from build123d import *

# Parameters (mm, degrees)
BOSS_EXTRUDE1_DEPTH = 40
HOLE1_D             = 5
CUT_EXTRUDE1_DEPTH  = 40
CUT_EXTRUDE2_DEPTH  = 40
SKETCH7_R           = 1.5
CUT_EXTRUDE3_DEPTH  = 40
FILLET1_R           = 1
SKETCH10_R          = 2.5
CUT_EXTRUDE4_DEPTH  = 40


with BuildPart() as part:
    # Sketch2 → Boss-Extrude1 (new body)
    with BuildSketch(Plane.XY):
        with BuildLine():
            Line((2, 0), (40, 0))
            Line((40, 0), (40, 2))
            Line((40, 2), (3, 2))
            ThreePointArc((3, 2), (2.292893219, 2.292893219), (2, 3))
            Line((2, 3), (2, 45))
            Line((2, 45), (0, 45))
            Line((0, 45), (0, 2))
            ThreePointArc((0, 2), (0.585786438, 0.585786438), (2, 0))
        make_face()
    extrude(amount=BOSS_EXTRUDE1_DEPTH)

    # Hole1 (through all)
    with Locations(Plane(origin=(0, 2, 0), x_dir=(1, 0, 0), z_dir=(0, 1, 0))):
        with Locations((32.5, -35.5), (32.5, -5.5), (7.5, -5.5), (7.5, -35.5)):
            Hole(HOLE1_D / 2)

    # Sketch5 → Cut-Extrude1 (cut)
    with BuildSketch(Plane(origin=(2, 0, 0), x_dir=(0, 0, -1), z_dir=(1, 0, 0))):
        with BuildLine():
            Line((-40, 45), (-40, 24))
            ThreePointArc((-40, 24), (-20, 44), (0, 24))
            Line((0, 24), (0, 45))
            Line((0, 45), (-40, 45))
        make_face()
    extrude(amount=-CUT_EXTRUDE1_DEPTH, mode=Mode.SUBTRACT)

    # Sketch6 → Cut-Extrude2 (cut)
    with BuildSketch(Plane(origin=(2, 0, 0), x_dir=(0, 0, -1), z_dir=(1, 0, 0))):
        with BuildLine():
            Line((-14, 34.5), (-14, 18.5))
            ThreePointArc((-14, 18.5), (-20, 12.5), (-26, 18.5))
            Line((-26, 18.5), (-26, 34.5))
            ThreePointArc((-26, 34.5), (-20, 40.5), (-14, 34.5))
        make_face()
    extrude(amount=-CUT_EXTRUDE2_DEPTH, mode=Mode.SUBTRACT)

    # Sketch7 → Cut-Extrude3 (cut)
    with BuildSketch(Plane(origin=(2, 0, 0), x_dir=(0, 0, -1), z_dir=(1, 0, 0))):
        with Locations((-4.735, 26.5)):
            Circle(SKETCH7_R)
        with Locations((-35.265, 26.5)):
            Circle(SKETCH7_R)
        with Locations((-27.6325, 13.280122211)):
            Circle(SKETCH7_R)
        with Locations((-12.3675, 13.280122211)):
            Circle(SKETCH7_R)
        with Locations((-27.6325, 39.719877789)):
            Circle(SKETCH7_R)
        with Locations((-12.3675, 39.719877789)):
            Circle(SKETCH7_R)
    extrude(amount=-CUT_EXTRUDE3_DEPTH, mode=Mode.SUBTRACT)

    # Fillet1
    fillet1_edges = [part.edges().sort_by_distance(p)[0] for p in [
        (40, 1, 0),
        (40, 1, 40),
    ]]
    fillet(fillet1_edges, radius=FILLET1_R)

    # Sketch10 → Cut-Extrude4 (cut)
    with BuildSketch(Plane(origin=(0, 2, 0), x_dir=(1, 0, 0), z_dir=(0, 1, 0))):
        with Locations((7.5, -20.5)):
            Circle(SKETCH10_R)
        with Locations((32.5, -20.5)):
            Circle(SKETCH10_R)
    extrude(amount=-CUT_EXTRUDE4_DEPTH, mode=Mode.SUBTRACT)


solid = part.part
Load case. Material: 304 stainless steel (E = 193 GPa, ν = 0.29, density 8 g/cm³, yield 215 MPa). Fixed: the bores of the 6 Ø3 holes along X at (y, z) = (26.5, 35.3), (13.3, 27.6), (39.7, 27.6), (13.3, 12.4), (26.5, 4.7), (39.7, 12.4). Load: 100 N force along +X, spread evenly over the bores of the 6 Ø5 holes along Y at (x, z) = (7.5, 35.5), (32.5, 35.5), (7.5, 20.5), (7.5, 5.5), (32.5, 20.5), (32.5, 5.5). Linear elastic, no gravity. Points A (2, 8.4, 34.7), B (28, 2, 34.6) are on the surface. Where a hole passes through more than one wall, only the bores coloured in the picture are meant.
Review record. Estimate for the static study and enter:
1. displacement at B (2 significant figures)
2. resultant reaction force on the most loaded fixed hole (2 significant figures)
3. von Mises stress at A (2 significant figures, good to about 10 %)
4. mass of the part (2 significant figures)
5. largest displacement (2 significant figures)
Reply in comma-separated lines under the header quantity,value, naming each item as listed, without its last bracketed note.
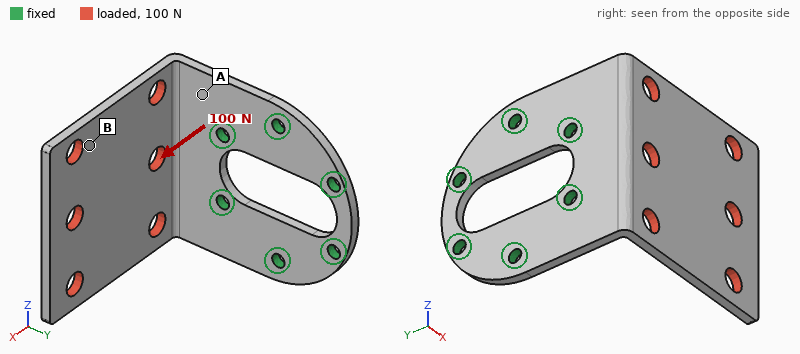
quantity,value
displacement at B,43 µm
resultant reaction force on the most loaded fixed hole,63 N
von Mises stress at A,24 MPa
mass of the part,42 g
largest displacement,62 µm
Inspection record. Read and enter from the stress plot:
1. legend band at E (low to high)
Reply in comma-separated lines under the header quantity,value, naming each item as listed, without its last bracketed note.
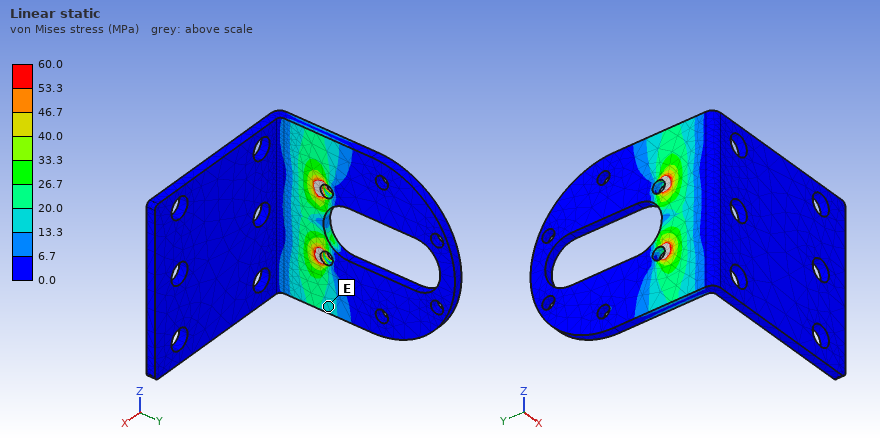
quantity,value
legend band at E,13.3 to 20.0 MPa
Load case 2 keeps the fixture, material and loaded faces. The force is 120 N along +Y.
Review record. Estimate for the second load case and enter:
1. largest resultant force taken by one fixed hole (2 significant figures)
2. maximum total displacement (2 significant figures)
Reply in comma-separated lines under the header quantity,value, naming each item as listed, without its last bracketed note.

quantity,value
largest resultant force taken by one fixed hole,59 N
maximum total displacement,0.39 mm
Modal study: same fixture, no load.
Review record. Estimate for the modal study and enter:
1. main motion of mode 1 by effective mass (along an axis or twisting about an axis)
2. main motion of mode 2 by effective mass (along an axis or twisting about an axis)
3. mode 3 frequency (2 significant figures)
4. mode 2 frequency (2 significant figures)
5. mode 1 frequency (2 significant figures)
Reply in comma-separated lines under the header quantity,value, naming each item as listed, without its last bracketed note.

quantity,value
main motion of mode 1 by effective mass,along Y
main motion of mode 2 by effective mass,along Z
mode 3 frequency,2500 Hz
mode 2 frequency,1600 Hz
mode 1 frequency,710 Hz
